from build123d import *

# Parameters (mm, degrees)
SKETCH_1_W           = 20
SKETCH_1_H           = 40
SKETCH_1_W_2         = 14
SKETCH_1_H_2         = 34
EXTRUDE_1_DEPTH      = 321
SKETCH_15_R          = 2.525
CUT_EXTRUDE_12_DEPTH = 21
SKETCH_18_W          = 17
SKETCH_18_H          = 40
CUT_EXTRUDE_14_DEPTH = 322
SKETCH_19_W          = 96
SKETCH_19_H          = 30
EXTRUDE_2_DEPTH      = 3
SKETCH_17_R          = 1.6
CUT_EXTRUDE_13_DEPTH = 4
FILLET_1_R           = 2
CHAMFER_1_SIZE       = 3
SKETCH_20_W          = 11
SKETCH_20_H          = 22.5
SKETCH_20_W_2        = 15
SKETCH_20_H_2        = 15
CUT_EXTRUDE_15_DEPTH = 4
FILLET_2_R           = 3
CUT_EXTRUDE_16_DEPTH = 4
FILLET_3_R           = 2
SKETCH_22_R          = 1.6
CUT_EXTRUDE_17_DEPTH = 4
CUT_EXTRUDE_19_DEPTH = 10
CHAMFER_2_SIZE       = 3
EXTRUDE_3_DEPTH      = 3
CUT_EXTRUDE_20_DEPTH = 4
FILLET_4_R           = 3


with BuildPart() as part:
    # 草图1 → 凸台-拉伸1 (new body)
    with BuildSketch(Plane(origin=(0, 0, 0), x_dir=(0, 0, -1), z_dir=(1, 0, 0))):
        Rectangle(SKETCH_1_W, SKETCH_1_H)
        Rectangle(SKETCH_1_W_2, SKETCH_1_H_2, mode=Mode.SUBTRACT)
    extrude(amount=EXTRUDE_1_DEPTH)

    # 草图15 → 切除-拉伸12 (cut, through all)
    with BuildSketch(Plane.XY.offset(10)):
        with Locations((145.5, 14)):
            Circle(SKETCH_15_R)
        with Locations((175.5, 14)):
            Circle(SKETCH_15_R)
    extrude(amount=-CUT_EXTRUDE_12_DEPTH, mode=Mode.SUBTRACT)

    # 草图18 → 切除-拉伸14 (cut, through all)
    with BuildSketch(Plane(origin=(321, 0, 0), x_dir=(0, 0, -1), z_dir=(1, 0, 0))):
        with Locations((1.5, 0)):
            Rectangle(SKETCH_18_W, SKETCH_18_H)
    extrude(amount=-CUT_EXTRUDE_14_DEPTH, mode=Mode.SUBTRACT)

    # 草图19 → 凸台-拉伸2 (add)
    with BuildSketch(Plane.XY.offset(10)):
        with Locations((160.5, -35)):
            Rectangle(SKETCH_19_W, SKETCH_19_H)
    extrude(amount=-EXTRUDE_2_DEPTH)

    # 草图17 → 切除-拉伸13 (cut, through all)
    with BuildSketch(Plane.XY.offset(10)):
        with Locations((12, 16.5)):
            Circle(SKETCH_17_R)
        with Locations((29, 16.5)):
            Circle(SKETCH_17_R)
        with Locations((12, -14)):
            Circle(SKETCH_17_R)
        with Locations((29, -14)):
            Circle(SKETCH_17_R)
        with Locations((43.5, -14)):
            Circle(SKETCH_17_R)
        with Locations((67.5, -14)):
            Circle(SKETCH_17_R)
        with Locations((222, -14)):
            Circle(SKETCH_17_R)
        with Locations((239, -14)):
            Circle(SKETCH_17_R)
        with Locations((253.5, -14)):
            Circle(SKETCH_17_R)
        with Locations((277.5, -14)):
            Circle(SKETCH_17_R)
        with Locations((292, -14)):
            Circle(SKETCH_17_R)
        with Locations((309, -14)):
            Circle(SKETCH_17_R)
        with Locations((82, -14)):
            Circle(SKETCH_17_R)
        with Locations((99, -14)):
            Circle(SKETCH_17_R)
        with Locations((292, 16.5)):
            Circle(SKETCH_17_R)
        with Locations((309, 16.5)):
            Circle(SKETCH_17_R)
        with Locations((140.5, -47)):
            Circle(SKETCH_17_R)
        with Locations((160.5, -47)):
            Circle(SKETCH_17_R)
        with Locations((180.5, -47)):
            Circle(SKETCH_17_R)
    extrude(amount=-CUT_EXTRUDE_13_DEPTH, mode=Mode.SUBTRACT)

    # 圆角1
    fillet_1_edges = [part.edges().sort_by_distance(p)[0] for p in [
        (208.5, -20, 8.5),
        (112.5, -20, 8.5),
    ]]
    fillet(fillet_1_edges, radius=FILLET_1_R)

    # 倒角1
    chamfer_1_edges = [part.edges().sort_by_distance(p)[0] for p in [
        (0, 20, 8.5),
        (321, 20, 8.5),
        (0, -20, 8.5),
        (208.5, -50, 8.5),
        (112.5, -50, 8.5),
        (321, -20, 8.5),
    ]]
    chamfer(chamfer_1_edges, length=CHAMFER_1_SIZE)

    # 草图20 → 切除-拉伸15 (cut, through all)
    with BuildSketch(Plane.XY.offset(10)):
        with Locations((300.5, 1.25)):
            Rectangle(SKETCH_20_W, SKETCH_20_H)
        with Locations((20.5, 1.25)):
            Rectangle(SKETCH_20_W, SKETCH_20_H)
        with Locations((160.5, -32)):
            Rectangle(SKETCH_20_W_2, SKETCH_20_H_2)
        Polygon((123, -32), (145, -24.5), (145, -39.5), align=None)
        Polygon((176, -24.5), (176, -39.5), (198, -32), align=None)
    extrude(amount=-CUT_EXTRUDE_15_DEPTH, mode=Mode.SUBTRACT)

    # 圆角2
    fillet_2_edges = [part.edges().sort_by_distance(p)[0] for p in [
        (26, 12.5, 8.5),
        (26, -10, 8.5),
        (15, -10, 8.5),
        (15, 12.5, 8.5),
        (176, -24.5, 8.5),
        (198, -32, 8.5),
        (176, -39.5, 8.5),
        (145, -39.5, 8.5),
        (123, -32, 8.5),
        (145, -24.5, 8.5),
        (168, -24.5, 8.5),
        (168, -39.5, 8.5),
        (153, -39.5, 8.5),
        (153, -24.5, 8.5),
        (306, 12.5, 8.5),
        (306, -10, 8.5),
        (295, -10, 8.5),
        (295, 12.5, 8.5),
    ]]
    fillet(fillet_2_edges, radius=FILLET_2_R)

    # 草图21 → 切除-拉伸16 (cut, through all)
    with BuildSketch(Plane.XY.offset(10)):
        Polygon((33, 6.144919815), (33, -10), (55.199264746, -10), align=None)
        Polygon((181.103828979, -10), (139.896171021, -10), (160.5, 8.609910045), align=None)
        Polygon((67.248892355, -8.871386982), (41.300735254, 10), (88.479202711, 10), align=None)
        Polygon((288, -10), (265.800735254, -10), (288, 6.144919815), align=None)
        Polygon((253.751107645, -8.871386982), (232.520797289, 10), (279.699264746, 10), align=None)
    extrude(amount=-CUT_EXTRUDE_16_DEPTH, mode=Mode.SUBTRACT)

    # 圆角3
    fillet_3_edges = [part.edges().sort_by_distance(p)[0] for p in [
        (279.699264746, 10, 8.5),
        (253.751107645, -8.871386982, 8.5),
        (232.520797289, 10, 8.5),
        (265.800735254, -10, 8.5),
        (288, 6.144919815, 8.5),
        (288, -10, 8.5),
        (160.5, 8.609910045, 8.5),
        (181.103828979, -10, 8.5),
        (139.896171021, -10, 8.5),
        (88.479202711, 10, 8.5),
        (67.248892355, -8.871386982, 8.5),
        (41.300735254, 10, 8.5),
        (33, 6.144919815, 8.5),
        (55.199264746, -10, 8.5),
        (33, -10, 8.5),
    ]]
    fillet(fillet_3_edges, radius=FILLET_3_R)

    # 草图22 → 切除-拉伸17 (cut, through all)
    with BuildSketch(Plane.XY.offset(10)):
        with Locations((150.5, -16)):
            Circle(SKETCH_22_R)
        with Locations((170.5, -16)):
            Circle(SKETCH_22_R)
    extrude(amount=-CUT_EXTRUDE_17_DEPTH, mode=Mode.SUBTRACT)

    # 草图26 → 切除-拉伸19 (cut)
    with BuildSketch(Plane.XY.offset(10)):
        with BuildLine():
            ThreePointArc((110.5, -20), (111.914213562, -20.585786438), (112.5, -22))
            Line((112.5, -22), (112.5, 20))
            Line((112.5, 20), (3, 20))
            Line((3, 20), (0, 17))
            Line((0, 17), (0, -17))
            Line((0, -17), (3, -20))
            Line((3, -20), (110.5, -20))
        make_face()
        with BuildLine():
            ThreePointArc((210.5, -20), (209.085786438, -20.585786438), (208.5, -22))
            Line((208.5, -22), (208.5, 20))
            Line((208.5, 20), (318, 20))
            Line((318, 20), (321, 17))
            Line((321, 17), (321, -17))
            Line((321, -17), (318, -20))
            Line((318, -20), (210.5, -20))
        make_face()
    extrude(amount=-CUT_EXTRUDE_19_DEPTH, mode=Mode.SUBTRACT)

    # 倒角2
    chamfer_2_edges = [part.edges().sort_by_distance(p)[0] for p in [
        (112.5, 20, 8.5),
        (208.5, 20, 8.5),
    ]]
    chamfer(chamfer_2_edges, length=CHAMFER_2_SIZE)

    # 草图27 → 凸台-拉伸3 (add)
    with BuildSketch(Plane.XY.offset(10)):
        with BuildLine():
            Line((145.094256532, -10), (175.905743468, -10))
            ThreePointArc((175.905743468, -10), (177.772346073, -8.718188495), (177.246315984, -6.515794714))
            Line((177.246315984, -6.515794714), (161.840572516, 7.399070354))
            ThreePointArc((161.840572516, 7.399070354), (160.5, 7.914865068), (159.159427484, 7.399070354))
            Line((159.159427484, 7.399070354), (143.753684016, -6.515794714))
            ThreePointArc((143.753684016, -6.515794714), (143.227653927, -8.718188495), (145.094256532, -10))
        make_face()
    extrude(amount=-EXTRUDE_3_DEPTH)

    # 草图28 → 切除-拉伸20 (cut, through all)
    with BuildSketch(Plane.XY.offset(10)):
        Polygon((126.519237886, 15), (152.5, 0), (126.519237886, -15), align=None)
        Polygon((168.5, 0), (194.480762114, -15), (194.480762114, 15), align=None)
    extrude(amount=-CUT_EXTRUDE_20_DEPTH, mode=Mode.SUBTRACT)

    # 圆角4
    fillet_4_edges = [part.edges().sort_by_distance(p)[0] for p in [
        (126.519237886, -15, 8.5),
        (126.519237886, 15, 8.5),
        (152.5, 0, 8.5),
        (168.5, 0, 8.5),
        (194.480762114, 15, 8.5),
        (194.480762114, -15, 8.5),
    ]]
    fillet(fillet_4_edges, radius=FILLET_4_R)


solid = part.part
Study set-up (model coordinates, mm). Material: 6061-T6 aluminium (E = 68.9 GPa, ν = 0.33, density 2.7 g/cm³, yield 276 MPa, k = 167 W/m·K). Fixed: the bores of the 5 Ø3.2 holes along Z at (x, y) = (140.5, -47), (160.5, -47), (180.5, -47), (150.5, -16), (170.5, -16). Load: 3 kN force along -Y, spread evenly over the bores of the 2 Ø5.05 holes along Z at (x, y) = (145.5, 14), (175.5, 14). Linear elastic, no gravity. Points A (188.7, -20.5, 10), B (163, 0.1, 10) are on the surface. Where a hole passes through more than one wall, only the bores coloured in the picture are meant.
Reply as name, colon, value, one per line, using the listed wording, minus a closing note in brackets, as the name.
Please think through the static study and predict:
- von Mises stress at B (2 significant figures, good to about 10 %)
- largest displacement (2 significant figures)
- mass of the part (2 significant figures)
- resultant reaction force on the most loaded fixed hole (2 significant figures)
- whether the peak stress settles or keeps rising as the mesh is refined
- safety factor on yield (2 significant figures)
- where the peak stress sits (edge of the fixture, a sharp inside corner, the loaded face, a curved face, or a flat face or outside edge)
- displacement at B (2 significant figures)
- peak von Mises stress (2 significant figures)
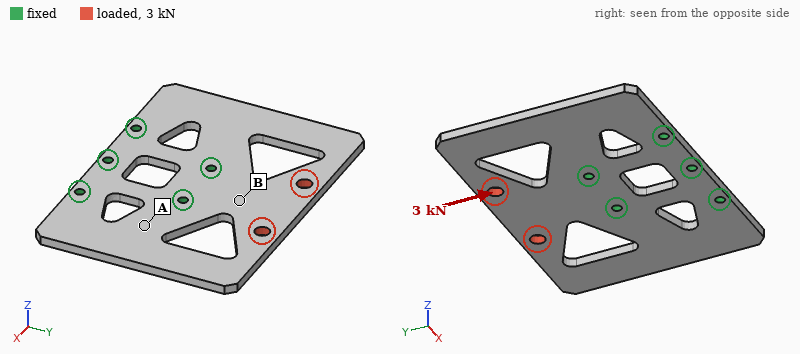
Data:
von Mises stress at B: 23 MPa
largest displacement: 29 µm
mass of the part: 44 g
resultant reaction force on the most loaded fixed hole: 1.4 kN
whether the peak stress settles or keeps rising as the mesh is refined: settles
safety factor on yield: 2.1
where the peak stress sits: a curved face
displacement at B: 8.6 µm
peak von Mises stress: 130 MPa
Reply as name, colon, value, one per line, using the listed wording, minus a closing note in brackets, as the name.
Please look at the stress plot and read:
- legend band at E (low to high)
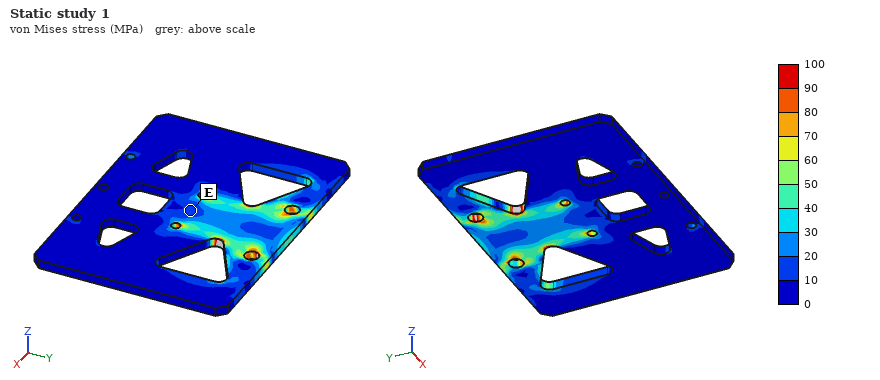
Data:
legend band at E: 10 to 20 MPa
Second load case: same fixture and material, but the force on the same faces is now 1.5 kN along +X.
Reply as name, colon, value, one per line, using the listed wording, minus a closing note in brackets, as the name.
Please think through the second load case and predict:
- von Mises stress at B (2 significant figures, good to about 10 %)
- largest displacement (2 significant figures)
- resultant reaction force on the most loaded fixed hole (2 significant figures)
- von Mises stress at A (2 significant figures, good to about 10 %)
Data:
von Mises stress at B: 34 MPa
largest displacement: 33 µm
resultant reaction force on the most loaded fixed hole: 1.3 kN
von Mises stress at A: 6.5 MPa
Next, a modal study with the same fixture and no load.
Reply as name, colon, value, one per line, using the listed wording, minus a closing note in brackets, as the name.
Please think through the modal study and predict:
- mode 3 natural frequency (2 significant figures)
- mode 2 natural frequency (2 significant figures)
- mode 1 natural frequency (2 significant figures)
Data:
mode 3 natural frequency: 2000 Hz
mode 2 natural frequency: 1200 Hz
mode 1 natural frequency: 1200 Hz
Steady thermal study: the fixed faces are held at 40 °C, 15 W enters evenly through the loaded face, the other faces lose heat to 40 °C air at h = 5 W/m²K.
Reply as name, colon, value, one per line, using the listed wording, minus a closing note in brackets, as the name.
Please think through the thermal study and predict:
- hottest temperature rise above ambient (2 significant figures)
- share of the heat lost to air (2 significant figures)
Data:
hottest temperature rise above ambient: 26 K
share of the heat lost to air: 3.2 %
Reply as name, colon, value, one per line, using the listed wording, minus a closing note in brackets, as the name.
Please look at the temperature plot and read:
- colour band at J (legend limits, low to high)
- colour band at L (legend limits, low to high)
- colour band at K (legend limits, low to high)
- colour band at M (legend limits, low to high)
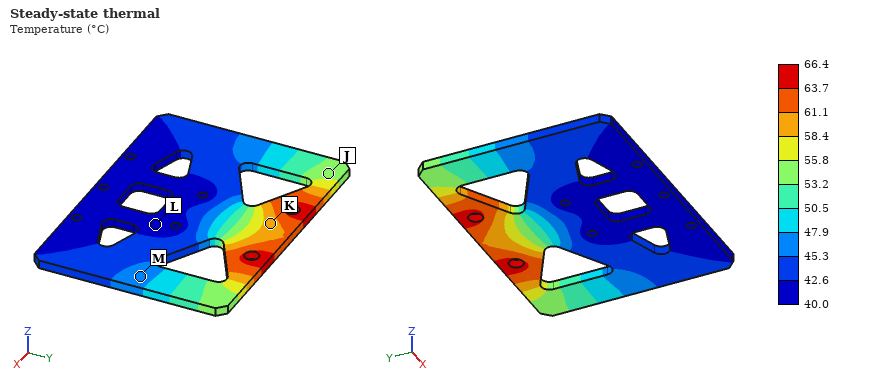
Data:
colour band at J: 53.2 to 55.8 °C
colour band at L: 40.0 to 42.6 °C
colour band at K: 58.4 to 61.1 °C
colour band at M: 45.3 to 47.9 °C
